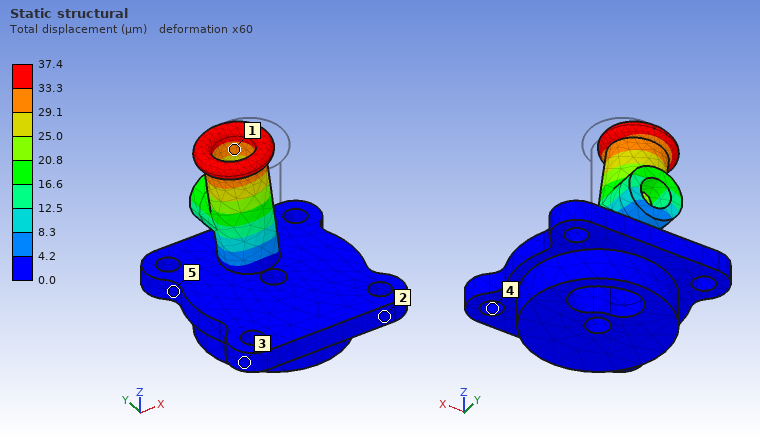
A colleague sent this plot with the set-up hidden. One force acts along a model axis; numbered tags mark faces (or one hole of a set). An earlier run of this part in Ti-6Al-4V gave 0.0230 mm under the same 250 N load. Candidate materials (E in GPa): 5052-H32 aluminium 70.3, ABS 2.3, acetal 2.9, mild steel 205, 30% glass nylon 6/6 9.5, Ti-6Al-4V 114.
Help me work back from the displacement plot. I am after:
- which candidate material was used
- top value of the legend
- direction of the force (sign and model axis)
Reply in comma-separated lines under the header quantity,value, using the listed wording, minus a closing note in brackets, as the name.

quantity,value
which candidate material was used,5052-H32 aluminium
top value of the legend,37.4 µm
direction of the force,-X
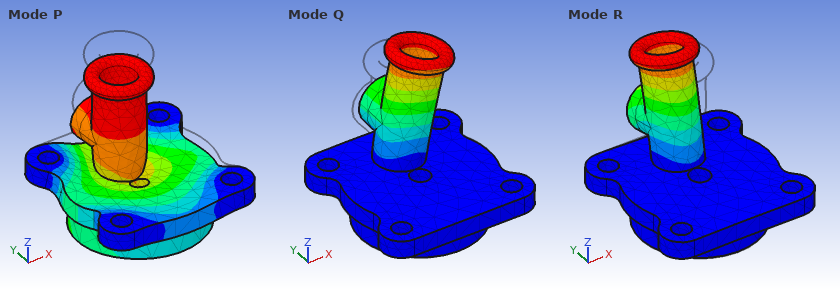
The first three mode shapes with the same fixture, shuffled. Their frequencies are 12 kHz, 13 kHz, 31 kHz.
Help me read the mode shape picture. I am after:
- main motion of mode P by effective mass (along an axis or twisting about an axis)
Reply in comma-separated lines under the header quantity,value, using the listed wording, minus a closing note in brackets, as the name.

quantity,value
main motion of mode P by effective mass,along Z
